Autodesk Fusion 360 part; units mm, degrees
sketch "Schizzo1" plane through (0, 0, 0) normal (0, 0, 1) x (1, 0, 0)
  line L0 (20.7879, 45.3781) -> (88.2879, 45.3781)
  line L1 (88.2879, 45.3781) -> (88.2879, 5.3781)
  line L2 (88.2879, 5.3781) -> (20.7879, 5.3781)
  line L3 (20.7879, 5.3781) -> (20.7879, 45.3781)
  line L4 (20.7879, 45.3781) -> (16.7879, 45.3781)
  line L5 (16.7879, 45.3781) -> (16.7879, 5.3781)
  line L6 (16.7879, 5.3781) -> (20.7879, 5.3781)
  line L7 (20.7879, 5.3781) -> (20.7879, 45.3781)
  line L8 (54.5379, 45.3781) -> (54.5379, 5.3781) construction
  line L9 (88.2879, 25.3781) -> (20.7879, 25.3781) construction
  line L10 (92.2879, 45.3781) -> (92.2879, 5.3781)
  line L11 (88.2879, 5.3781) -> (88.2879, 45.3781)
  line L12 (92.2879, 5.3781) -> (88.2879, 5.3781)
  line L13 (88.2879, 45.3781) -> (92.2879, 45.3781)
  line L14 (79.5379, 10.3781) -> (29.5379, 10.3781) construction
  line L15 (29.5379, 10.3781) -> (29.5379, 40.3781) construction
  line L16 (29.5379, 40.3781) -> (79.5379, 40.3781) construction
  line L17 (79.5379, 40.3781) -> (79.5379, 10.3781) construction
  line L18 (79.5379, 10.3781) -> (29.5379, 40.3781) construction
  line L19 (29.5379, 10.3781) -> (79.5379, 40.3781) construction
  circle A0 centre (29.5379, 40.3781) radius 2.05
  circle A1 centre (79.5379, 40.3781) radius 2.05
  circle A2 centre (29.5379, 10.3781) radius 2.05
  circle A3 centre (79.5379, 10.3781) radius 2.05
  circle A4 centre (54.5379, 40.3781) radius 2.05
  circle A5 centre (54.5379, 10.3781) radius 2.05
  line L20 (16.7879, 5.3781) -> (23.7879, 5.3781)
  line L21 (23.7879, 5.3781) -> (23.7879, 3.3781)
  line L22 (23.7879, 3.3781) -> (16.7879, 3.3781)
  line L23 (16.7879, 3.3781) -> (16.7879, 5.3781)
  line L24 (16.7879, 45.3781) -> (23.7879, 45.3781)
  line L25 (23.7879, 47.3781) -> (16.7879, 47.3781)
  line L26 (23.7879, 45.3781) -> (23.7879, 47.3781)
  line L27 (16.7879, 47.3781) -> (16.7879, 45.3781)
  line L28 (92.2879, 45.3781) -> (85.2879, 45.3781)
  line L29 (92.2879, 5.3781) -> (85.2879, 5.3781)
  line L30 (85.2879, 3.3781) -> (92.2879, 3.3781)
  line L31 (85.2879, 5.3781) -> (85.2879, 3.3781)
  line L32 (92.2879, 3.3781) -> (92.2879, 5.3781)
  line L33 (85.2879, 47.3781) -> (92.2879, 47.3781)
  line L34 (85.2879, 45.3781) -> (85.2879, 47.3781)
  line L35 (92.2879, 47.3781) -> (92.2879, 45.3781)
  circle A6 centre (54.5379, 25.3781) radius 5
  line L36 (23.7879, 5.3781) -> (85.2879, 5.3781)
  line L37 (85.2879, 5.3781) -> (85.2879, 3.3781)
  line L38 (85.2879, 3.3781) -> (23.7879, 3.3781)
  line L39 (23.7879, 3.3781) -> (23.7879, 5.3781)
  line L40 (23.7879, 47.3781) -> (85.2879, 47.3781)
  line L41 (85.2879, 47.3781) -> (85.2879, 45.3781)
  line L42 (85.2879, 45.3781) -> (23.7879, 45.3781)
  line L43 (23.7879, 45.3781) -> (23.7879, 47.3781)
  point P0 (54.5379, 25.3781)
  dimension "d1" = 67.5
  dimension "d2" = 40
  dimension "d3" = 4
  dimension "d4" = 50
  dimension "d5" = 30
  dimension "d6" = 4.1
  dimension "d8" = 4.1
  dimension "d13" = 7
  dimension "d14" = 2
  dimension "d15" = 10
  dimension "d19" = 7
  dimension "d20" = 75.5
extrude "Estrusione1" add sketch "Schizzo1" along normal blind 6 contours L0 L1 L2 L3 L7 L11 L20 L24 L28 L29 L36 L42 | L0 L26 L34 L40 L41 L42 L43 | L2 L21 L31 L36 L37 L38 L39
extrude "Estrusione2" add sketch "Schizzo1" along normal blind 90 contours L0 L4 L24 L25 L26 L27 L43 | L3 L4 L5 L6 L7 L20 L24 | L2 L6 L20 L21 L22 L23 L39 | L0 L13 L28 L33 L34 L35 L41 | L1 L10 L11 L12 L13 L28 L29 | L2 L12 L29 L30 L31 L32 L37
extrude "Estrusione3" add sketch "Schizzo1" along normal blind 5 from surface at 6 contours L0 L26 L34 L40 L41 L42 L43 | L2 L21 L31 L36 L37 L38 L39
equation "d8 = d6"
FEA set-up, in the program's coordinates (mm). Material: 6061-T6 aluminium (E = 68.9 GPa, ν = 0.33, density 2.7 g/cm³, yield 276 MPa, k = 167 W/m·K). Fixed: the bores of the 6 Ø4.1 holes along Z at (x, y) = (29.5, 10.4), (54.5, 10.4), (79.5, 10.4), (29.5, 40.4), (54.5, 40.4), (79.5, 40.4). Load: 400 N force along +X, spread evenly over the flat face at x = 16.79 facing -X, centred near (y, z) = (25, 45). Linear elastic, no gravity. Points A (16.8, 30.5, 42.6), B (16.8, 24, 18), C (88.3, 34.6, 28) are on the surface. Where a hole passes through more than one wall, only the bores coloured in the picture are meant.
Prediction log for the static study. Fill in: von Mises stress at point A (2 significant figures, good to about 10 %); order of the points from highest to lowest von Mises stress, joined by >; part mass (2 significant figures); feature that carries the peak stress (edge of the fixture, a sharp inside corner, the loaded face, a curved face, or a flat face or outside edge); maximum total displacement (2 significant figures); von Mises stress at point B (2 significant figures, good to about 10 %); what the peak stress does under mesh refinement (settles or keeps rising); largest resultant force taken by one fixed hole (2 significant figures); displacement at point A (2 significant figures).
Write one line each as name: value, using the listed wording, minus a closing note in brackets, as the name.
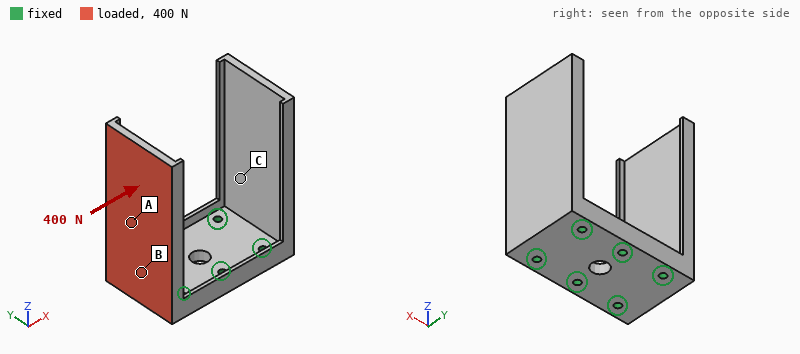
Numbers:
von Mises stress at point A: 30 MPa
order of the points from highest to lowest von Mises stress, joined by >: B > A > C
part mass: 140 g
feature that carries the peak stress: a sharp inside corner
maximum total displacement: 1.2 mm
von Mises stress at point B: 53 MPa
what the peak stress does under mesh refinement: keeps rising
largest resultant force taken by one fixed hole: 210 N
displacement at point A: 0.39 mm
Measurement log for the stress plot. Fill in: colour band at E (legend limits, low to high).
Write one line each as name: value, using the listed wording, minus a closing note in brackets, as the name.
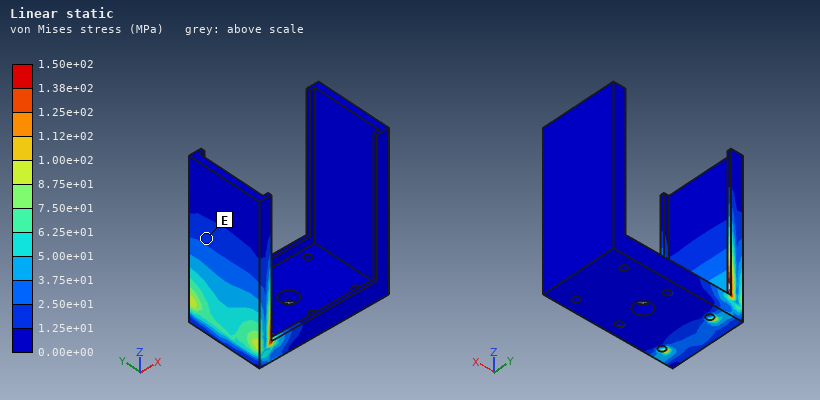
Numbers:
colour band at E: 1.25e+01 to 2.50e+01 MPa
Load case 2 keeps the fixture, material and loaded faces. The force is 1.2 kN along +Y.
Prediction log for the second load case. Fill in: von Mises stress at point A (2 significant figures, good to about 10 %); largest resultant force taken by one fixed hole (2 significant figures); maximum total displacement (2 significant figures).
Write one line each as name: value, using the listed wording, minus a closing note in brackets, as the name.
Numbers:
von Mises stress at point A: 12 MPa
largest resultant force taken by one fixed hole: 1.8 kN
maximum total displacement: 0.16 mm
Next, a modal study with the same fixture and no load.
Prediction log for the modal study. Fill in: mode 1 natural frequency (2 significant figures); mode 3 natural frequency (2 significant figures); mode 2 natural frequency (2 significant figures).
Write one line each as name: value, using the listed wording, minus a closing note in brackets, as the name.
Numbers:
mode 1 natural frequency: 530 Hz
mode 3 natural frequency: 1800 Hz
mode 2 natural frequency: 530 Hz
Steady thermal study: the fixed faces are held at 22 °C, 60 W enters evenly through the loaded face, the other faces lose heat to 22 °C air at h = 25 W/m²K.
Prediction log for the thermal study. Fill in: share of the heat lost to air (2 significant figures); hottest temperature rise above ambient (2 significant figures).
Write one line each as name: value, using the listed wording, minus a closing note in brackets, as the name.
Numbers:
share of the heat lost to air: 14 %
hottest temperature rise above ambient: 76 K
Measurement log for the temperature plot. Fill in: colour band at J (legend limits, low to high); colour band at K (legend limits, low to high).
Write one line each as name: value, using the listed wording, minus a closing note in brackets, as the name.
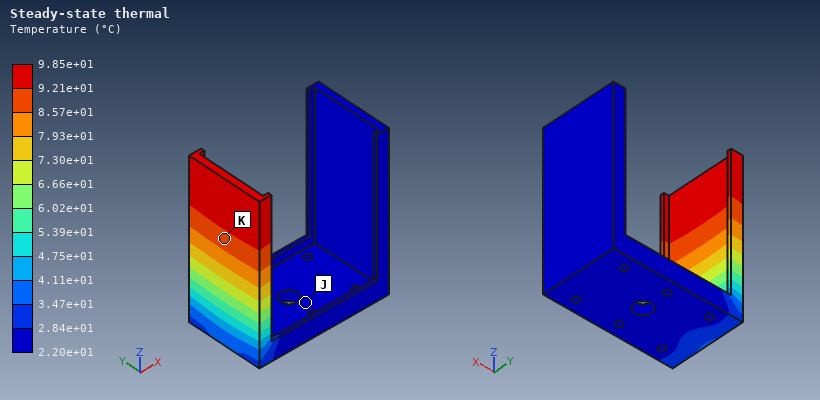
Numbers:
colour band at J: 2.20e+01 to 2.84e+01 °C
colour band at K: 8.57e+01 to 9.21e+01 °C
